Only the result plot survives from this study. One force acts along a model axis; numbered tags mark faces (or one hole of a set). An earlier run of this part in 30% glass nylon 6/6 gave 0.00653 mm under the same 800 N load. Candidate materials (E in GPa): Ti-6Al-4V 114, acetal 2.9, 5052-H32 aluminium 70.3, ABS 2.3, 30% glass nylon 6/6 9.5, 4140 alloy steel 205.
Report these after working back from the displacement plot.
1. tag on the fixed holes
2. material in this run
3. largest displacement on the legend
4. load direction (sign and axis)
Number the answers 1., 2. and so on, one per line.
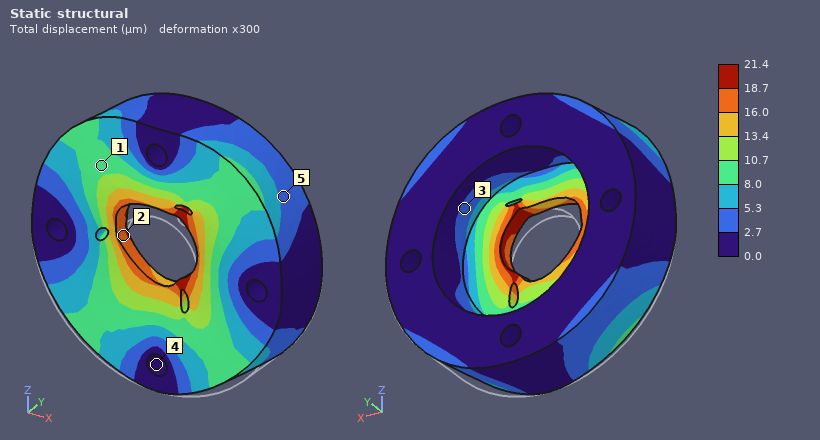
1. 4
2. acetal
3. 21.4 µm
4. +Z
